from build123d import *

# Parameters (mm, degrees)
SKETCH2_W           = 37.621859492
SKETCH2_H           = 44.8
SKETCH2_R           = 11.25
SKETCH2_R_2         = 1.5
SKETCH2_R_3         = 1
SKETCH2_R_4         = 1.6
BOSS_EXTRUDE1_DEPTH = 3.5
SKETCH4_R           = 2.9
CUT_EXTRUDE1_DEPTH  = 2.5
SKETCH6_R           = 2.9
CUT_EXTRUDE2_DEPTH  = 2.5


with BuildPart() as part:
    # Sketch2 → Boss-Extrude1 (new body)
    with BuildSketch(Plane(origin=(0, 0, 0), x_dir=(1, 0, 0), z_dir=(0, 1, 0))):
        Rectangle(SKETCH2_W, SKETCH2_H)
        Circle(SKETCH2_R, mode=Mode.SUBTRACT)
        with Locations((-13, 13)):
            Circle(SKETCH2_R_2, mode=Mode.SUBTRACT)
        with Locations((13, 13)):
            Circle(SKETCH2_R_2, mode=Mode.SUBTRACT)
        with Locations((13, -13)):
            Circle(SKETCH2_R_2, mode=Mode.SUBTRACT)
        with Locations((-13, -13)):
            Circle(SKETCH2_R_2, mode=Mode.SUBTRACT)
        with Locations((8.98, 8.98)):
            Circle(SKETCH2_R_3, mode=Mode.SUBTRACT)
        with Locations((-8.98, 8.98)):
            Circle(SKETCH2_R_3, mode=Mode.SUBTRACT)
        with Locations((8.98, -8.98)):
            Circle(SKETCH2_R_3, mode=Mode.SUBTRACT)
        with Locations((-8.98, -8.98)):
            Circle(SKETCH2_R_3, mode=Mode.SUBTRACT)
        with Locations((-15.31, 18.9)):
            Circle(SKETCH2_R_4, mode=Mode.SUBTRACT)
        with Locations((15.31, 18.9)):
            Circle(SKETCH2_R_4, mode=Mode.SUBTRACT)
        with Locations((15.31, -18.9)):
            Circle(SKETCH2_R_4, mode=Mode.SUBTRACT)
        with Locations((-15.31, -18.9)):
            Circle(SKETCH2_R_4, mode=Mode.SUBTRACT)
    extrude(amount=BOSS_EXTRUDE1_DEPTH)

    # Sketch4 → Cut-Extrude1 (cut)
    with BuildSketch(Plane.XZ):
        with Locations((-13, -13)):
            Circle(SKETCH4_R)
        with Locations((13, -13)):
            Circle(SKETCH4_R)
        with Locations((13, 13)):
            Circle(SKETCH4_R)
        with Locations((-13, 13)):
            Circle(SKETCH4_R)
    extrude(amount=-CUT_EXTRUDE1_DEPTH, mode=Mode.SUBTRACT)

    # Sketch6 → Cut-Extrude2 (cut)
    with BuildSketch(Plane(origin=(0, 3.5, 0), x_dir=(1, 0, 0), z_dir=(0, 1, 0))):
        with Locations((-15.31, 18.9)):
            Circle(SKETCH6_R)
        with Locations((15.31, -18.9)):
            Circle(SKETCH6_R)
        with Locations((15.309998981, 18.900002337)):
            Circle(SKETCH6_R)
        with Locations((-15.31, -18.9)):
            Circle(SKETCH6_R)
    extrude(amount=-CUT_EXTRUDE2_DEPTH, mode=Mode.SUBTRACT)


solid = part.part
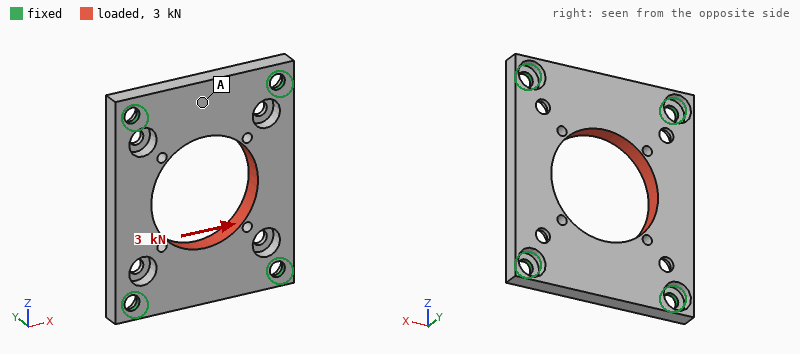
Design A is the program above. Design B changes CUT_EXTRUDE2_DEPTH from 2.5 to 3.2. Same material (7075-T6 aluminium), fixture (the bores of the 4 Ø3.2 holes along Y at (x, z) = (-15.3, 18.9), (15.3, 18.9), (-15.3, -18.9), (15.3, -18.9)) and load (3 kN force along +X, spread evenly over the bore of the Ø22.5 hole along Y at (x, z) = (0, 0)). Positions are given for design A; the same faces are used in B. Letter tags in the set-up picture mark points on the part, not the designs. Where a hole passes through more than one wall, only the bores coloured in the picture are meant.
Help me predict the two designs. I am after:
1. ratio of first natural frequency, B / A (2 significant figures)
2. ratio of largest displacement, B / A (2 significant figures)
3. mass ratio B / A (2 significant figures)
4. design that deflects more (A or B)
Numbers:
0.75
1.5
0.99
B
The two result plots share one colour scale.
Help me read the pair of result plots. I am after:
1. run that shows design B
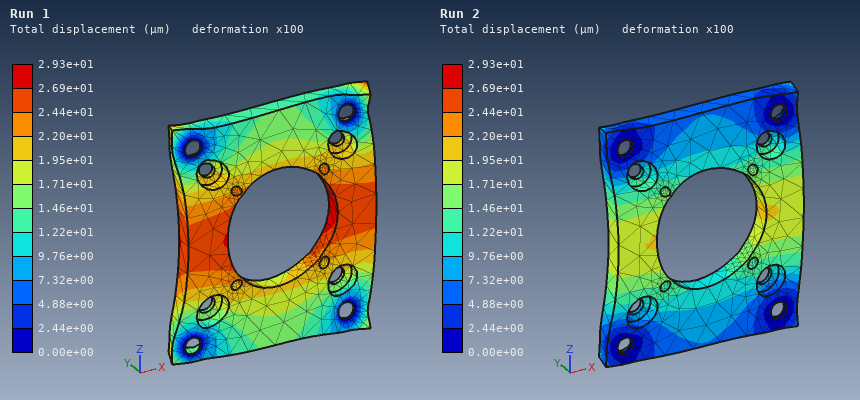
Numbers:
Run 1
